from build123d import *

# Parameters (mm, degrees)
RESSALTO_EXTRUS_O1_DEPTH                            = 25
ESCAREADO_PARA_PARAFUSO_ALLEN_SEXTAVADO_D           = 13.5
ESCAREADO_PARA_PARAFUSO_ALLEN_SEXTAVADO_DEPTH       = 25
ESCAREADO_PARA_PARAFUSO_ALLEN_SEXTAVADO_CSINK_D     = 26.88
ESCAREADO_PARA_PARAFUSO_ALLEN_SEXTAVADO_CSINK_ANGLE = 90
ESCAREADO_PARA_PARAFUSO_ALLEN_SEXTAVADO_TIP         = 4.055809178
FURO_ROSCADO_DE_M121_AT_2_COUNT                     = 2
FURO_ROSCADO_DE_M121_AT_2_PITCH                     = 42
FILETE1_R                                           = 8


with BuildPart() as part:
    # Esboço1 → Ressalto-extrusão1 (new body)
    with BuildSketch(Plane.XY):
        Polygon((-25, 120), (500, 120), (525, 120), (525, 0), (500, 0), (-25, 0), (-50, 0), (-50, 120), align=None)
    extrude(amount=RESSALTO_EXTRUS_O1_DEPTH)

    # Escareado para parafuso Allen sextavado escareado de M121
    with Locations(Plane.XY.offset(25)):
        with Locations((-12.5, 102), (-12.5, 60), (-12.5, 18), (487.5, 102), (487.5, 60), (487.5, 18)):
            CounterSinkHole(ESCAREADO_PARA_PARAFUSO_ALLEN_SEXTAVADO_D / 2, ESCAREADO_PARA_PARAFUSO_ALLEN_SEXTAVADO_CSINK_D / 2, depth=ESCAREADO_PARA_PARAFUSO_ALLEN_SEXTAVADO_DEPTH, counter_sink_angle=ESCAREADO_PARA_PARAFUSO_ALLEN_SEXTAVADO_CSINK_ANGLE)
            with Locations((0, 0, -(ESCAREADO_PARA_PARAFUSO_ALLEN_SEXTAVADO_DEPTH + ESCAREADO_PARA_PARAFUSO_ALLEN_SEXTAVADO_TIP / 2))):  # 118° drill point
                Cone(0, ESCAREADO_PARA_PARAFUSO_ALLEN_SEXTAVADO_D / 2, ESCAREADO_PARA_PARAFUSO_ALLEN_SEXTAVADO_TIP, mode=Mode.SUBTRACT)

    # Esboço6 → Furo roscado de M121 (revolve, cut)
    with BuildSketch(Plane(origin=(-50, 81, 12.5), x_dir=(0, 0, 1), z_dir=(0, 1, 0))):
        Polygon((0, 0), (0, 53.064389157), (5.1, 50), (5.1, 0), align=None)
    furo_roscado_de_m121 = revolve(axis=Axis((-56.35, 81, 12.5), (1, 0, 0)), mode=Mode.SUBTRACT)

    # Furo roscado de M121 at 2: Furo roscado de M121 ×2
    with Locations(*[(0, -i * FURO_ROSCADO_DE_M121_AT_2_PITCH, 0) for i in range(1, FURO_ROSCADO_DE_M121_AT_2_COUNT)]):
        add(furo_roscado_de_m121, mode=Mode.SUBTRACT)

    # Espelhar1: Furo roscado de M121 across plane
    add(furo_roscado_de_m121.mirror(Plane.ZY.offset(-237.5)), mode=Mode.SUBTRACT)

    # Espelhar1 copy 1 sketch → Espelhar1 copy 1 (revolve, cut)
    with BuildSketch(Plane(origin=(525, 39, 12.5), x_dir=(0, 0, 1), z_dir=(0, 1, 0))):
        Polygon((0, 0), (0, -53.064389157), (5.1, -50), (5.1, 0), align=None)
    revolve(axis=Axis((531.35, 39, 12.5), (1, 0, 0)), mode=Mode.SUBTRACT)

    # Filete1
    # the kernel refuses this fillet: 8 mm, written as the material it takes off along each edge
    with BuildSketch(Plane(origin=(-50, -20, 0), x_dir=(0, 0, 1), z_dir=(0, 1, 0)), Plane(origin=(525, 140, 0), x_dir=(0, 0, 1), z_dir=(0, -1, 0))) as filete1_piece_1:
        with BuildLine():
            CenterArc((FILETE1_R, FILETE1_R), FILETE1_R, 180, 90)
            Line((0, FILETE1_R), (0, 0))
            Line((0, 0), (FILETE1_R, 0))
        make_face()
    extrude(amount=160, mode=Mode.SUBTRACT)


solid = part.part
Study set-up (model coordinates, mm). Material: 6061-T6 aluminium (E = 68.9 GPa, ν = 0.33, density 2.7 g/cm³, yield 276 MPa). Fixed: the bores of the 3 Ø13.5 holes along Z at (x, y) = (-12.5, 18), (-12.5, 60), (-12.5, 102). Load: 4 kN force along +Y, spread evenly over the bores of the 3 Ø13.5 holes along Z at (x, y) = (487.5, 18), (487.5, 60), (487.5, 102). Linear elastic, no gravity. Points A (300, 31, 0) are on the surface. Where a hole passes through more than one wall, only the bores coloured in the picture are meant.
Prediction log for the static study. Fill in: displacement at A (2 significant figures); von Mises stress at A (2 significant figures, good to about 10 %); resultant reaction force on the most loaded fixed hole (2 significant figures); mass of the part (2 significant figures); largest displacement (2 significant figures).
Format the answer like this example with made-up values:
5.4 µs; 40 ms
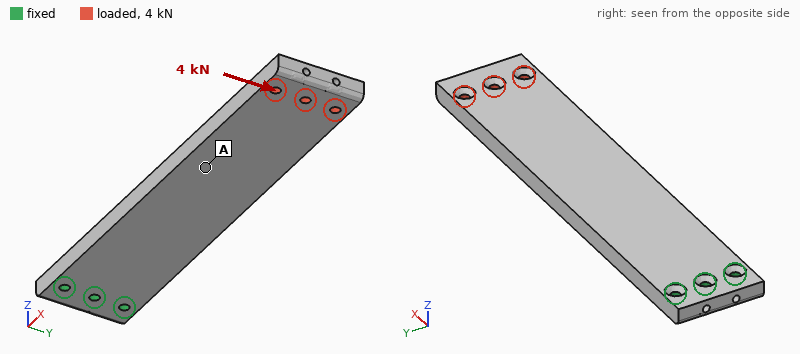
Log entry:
0.35 mm; 7.1 MPa; 22 kN; 4.5 kg; 0.81 mm
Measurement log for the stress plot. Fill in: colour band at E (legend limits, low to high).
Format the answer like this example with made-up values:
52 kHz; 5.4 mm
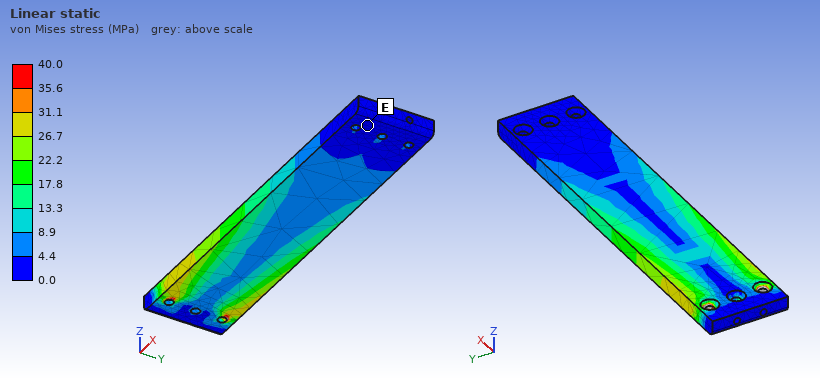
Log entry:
0.0 to 4.4 MPa
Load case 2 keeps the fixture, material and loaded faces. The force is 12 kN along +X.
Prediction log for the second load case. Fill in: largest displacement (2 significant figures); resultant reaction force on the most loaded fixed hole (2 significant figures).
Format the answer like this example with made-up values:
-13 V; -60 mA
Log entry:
0.52 mm; 4.1 kN
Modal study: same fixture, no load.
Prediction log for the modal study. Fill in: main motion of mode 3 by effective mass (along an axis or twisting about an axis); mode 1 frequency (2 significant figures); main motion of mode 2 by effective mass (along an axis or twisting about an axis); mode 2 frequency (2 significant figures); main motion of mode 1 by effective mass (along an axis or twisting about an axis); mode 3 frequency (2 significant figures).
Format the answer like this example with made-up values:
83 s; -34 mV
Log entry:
along Z; 71 Hz; along Y; 330 Hz; along Z; 440 Hz
